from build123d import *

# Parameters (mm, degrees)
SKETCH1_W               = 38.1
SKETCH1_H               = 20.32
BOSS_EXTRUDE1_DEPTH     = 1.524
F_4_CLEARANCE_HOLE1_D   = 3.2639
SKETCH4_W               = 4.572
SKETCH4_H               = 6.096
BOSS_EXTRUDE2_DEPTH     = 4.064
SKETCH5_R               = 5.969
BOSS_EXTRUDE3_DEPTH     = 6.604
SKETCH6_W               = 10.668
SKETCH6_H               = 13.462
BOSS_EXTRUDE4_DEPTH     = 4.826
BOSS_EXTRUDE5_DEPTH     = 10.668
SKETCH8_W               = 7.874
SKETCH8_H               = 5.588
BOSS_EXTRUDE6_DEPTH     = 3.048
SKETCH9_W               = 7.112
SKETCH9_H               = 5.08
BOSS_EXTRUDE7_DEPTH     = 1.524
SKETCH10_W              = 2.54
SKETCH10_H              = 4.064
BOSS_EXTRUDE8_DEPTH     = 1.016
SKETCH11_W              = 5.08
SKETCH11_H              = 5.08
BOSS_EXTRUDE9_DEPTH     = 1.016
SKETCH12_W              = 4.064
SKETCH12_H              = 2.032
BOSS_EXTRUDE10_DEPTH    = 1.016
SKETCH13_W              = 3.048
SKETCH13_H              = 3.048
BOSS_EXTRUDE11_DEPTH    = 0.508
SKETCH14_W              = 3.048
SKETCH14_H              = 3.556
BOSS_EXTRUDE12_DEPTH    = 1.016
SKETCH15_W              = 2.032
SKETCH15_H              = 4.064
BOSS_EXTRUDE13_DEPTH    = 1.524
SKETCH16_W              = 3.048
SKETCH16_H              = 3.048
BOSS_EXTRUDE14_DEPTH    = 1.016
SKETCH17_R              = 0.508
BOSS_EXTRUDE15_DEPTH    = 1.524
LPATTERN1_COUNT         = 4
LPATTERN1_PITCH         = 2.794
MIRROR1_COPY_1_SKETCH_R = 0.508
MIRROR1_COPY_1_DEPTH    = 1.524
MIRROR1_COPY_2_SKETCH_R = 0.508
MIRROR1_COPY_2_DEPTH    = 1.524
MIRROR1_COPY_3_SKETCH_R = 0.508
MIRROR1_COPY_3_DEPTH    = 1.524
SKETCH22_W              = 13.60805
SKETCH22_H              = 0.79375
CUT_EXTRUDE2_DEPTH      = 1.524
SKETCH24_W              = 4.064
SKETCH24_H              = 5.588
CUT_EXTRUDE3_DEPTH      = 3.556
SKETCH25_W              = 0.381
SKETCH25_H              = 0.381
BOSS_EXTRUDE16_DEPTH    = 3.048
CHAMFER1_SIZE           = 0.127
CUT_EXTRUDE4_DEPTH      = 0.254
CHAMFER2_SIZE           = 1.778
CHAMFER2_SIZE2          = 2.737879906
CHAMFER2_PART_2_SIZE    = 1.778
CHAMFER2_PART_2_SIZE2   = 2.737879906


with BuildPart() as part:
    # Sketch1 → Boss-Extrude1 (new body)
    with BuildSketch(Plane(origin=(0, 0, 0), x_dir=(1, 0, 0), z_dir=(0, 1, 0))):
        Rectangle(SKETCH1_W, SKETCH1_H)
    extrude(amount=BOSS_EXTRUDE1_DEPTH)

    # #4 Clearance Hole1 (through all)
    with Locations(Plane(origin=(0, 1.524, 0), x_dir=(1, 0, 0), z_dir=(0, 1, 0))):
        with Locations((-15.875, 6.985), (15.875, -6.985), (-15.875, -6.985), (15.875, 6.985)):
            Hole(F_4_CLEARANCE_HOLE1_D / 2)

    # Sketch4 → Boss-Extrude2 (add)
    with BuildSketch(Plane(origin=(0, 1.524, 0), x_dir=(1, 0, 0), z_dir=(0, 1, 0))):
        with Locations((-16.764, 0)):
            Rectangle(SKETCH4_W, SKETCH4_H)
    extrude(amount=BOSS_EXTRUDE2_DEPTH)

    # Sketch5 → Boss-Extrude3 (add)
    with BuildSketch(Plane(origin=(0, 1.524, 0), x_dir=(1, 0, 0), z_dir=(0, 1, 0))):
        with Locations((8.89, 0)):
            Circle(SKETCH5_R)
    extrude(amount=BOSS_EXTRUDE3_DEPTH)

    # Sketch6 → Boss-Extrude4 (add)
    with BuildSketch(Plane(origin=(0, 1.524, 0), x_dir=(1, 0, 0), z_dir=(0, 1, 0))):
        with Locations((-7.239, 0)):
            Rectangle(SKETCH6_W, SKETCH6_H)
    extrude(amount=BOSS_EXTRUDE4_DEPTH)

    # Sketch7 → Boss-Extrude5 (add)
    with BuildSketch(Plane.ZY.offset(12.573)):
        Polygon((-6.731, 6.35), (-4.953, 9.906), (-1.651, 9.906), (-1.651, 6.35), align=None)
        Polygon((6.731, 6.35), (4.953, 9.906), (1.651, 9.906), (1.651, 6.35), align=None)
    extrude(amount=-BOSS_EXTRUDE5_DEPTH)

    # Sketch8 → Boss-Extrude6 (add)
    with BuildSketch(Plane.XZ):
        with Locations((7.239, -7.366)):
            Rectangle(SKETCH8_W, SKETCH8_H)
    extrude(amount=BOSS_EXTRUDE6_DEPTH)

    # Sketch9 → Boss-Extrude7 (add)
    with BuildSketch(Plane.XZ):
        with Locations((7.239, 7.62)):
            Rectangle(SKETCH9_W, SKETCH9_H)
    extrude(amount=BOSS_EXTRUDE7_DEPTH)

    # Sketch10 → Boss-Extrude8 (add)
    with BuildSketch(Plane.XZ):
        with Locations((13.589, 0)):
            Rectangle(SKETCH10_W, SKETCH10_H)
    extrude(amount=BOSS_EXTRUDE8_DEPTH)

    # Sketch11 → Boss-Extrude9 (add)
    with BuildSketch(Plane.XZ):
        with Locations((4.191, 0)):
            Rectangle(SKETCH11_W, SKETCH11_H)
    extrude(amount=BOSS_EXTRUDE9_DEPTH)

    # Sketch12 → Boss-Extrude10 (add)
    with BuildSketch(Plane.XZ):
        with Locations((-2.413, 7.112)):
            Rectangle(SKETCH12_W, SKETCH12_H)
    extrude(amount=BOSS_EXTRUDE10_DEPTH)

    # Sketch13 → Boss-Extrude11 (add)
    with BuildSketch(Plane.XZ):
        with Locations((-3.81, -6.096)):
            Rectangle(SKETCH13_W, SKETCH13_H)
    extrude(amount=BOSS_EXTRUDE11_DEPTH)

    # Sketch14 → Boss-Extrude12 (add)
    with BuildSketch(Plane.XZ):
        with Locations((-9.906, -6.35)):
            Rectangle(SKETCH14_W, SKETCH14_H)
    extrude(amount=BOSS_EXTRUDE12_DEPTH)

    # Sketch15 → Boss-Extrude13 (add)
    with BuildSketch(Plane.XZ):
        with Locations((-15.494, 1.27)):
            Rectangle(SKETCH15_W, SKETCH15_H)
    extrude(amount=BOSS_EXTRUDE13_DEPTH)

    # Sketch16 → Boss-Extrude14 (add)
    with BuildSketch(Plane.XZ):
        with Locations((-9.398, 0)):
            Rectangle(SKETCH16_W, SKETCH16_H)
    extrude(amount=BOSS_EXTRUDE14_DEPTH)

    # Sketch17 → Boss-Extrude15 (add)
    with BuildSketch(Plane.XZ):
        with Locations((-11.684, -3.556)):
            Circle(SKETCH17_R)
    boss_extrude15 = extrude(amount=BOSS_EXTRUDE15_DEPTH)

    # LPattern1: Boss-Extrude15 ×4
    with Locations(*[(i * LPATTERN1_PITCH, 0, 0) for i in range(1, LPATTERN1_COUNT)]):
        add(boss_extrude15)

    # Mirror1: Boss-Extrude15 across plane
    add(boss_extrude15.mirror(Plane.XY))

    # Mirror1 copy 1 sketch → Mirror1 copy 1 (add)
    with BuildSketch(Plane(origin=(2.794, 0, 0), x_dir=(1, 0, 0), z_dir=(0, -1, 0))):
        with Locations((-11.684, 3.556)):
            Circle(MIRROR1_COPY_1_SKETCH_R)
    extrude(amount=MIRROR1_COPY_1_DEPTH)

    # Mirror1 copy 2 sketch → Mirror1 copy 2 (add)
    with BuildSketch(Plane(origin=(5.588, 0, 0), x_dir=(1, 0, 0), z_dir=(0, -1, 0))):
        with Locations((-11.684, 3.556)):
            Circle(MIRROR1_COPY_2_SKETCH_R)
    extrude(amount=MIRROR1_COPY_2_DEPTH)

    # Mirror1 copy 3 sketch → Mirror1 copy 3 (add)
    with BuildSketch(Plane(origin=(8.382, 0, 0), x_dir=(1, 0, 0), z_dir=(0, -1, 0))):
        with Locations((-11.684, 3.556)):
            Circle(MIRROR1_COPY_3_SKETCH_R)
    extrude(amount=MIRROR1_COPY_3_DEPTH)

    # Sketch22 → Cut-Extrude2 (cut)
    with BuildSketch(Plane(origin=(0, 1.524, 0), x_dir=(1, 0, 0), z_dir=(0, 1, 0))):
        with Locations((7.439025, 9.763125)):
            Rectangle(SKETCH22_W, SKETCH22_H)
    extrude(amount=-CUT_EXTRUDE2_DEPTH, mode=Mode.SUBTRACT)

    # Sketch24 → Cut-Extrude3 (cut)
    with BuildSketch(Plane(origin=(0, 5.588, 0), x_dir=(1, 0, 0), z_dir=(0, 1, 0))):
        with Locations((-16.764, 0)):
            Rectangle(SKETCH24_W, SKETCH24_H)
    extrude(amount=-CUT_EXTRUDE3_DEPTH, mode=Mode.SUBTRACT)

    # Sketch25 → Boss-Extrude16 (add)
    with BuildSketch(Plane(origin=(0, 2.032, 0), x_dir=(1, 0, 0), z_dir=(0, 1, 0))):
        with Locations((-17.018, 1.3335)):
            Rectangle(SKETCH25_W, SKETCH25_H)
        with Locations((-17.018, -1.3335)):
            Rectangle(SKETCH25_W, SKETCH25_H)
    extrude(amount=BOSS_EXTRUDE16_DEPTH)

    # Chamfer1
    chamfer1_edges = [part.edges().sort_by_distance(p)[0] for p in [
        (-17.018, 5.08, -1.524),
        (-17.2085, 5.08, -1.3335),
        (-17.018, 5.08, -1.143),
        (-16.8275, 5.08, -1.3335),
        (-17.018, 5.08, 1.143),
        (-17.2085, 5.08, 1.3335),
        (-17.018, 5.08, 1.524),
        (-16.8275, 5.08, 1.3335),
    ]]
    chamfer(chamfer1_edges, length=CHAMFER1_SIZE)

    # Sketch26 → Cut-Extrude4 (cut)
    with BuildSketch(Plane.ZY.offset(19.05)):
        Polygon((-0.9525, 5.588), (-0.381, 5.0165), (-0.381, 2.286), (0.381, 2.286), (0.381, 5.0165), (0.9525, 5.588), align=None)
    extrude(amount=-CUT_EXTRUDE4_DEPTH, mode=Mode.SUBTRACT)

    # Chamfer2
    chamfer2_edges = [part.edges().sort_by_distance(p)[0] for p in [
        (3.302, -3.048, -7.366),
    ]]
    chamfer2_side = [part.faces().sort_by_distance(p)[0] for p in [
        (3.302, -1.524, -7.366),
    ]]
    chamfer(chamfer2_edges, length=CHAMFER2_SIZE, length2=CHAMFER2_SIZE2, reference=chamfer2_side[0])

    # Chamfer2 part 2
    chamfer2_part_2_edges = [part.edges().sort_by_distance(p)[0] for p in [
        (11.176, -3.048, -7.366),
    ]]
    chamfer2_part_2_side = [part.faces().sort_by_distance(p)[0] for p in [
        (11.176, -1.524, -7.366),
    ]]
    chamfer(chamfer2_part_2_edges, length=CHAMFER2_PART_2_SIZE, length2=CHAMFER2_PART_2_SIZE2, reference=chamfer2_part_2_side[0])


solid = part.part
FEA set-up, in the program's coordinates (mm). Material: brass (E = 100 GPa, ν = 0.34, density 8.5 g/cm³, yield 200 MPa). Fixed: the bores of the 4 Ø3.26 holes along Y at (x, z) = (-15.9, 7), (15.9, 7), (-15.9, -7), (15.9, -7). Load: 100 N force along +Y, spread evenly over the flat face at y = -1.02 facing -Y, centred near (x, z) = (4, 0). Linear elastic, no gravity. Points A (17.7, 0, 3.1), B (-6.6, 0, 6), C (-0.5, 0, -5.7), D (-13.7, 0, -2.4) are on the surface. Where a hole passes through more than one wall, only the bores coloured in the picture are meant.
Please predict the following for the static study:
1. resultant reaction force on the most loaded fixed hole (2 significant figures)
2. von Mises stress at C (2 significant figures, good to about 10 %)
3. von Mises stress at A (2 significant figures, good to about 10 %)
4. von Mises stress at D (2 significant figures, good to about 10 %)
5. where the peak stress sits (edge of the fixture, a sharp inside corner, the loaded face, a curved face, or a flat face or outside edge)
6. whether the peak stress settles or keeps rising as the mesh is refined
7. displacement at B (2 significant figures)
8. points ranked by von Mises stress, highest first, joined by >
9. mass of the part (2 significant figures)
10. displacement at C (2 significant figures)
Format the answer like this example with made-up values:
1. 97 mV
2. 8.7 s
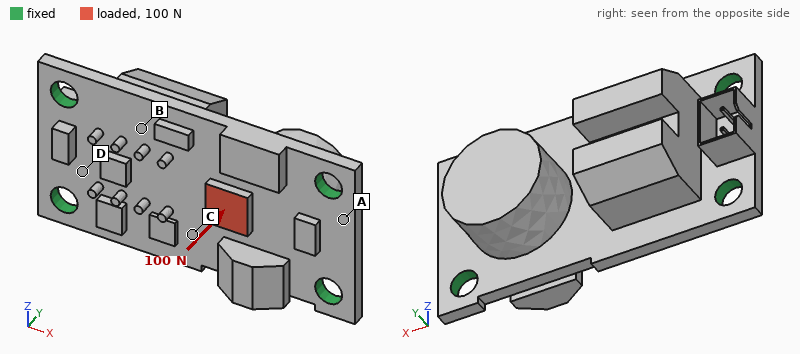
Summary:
1. 36 N
2. 22 MPa
3. 7.6 MPa
4. 16 MPa
5. edge of the fixture
6. keeps rising
7. 7.6 µm
8. C > D > A > B
9. 27 g
10. 13 µm
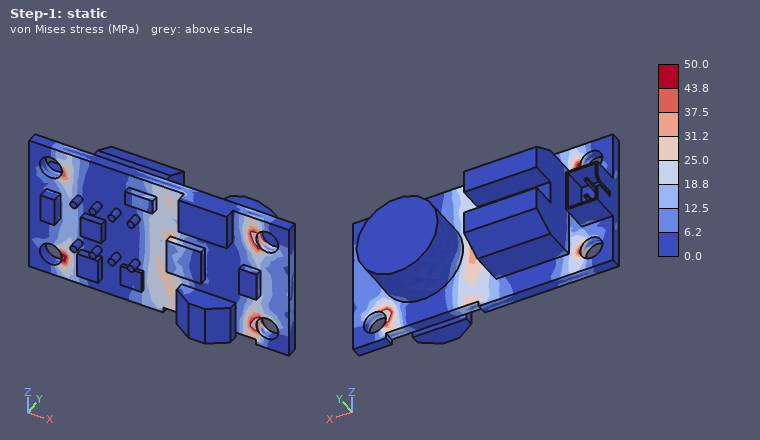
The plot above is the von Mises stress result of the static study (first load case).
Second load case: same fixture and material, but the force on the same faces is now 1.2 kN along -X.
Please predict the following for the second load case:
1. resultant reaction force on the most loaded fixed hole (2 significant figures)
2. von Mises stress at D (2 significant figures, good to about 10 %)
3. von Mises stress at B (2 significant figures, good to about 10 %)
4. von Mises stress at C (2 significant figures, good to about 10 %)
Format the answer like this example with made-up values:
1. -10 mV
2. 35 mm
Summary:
1. 380 N
2. 30 MPa
3. 19 MPa
4. 63 MPa
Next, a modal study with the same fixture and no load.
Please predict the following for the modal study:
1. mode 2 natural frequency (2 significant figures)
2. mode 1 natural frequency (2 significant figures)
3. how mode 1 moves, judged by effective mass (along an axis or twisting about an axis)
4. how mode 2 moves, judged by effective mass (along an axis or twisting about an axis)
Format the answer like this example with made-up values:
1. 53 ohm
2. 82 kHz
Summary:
1. 12 kHz
2. 3800 Hz
3. along Y
4. along Z
